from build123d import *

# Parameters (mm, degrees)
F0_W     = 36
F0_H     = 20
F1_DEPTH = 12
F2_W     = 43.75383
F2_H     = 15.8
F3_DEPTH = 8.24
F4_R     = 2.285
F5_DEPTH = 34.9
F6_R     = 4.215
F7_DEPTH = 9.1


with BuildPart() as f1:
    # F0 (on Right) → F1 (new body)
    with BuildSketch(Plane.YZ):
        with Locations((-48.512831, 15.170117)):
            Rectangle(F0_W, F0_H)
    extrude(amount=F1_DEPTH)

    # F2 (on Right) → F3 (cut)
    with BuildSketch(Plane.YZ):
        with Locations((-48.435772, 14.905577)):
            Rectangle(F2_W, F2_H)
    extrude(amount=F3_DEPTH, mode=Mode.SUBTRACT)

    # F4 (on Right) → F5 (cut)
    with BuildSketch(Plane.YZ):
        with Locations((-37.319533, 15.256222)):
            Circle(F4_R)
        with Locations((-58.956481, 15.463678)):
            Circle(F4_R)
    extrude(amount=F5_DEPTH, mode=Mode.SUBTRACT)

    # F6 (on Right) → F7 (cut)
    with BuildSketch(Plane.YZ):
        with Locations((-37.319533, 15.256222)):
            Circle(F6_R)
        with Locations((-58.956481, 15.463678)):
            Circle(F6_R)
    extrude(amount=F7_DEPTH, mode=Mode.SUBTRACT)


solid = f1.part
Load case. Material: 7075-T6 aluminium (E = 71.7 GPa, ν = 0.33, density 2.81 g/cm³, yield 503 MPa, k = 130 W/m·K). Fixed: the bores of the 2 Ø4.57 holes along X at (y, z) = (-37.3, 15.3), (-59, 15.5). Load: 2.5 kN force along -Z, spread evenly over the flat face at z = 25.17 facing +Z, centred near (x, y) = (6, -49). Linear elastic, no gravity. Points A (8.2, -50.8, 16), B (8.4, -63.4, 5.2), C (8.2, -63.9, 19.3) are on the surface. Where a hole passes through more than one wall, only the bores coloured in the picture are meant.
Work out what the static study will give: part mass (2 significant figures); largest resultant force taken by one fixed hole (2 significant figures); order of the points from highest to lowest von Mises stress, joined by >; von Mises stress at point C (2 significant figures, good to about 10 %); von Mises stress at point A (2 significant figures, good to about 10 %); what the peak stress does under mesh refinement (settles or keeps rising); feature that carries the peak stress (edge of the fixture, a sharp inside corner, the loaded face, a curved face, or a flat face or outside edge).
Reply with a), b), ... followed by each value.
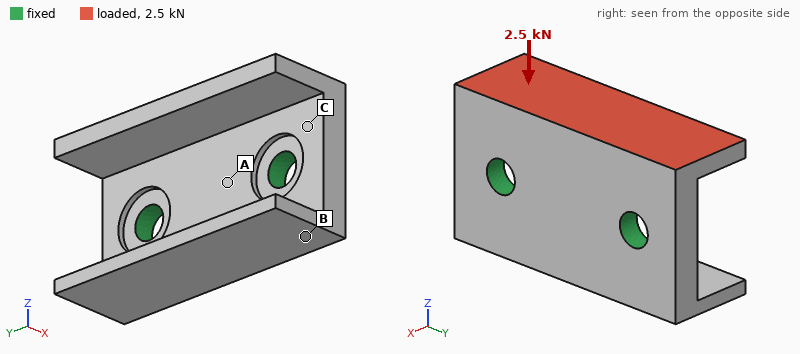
a) 11 g
b) 1.3 kN
c) C > A > B
d) 140 MPa
e) 80 MPa
f) keeps rising
g) edge of the fixture
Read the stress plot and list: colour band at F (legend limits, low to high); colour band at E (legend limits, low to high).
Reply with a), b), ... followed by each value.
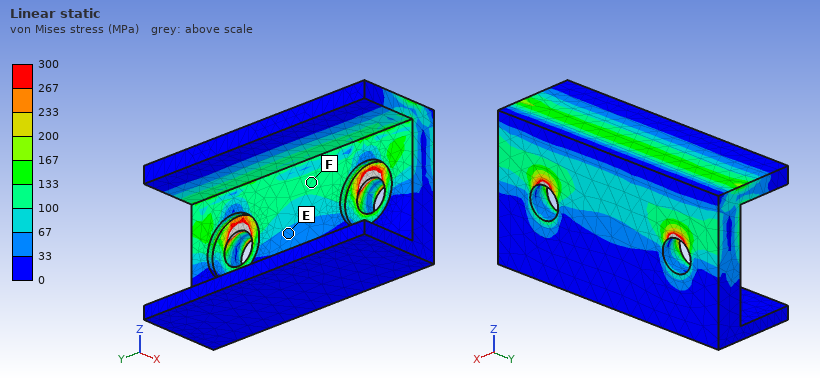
a) 100 to 133 MPa
b) 33 to 67 MPa
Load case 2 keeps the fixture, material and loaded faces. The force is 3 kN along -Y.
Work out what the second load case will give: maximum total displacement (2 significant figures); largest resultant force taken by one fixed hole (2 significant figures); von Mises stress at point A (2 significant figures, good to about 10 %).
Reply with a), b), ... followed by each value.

a) 44 µm
b) 2.0 kN
c) 42 MPa
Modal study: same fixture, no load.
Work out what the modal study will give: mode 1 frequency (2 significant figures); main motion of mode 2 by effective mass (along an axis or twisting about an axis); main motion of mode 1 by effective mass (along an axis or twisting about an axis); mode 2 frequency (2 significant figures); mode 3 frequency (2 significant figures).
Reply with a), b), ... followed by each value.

a) 11 kHz
b) along X
c) along Z
d) 13 kHz
e) 15 kHz
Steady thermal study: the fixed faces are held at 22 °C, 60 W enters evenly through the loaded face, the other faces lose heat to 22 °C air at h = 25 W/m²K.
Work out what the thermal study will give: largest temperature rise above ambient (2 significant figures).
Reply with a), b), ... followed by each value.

a) 52 K
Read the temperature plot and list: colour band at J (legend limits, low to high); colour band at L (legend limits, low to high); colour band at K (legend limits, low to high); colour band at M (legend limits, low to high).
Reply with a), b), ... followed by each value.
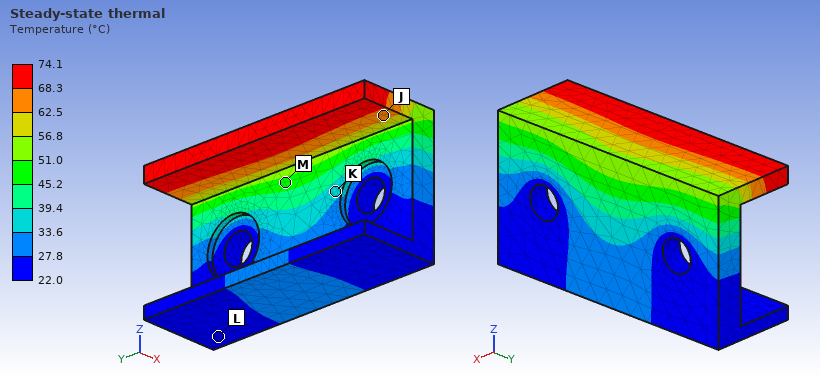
a) 62.5 to 68.3 °C
b) 22.0 to 27.8 °C
c) 33.6 to 39.4 °C
d) 45.2 to 51.0 °C
